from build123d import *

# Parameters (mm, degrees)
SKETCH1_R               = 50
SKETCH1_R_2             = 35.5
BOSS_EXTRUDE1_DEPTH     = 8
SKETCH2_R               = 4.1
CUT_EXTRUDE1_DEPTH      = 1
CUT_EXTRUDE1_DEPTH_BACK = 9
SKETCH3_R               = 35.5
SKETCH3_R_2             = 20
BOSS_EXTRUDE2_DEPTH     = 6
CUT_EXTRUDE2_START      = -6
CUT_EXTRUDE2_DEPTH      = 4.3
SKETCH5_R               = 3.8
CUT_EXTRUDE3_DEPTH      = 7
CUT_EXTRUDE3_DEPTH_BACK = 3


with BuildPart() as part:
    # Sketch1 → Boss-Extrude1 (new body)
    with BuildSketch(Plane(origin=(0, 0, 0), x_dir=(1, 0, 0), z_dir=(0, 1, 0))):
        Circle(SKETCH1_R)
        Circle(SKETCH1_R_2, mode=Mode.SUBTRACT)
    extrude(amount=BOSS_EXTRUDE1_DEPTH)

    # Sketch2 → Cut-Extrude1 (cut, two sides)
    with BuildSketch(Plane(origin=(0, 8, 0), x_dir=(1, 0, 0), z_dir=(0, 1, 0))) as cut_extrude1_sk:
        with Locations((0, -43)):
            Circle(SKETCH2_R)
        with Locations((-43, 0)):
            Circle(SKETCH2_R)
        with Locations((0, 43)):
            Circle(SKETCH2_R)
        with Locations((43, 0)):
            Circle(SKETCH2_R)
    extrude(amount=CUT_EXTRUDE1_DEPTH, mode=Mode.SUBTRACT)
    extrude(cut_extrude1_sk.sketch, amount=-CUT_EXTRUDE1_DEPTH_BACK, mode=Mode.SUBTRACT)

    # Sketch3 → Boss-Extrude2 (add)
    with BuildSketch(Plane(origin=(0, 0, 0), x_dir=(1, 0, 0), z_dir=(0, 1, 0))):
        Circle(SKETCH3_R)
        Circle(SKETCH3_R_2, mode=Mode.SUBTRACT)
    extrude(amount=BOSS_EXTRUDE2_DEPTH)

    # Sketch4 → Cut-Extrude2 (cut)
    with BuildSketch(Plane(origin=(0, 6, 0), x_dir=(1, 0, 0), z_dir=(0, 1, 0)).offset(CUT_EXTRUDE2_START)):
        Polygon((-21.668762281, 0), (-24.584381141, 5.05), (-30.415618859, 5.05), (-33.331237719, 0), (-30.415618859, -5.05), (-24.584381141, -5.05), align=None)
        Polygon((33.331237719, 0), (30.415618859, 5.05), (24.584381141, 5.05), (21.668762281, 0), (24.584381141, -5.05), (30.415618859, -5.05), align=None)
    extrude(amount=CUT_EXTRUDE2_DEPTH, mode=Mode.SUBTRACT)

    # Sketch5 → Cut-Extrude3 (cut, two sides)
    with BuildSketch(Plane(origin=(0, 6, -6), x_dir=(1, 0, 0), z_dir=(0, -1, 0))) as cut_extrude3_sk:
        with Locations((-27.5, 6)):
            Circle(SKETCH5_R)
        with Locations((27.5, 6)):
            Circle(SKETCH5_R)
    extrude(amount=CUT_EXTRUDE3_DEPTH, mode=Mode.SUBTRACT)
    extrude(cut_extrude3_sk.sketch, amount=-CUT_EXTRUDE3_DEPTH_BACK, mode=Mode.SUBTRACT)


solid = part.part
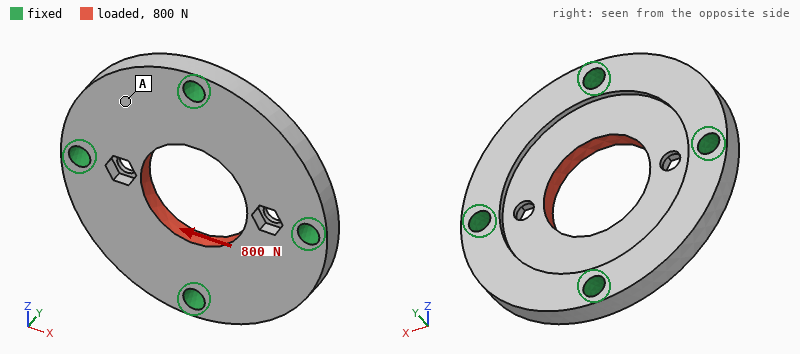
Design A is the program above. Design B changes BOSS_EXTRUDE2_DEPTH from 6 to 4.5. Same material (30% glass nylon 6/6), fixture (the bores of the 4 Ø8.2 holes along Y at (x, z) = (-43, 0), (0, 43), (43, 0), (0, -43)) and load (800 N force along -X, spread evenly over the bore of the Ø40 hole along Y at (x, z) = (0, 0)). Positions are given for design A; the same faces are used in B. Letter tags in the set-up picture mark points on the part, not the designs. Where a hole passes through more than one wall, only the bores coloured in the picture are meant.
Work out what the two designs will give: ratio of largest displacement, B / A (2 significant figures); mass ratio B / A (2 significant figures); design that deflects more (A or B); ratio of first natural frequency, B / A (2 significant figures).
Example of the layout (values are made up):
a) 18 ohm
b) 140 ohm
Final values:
a) 1.4
b) 0.91
c) B
d) 1.00
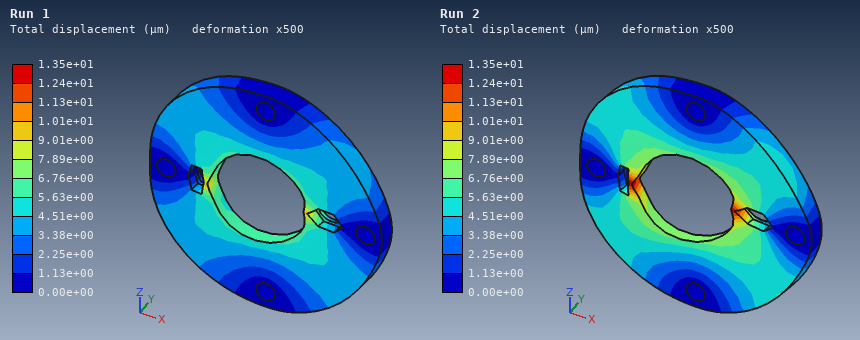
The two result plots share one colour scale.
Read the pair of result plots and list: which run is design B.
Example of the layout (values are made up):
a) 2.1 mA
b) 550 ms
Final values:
a) Run 2
